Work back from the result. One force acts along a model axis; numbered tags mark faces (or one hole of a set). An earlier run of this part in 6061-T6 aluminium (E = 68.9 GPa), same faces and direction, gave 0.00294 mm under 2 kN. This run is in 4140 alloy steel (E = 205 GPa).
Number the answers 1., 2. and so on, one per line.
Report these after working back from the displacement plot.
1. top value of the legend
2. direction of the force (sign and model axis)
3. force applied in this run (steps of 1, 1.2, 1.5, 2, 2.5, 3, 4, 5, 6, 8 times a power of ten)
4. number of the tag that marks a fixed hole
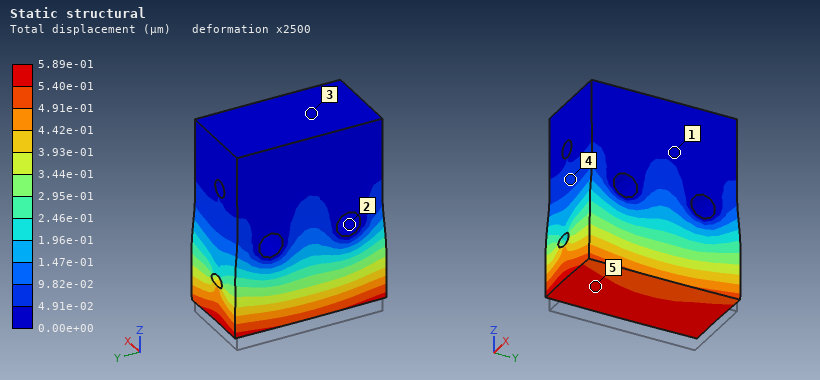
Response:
1. 5.89e-01 µm
2. +Z
3. 1.2 kN
4. 2
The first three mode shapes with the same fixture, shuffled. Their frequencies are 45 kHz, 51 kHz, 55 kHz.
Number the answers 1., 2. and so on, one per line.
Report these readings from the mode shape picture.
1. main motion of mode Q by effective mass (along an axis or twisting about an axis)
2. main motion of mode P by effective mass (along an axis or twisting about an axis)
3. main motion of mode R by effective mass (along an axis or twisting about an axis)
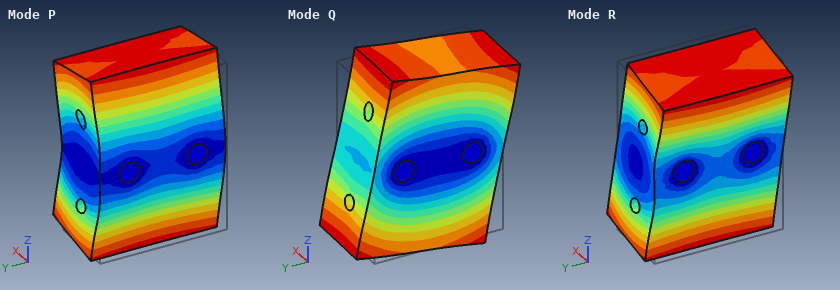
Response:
1. twisting about X
2. along X
3. twisting about Y
